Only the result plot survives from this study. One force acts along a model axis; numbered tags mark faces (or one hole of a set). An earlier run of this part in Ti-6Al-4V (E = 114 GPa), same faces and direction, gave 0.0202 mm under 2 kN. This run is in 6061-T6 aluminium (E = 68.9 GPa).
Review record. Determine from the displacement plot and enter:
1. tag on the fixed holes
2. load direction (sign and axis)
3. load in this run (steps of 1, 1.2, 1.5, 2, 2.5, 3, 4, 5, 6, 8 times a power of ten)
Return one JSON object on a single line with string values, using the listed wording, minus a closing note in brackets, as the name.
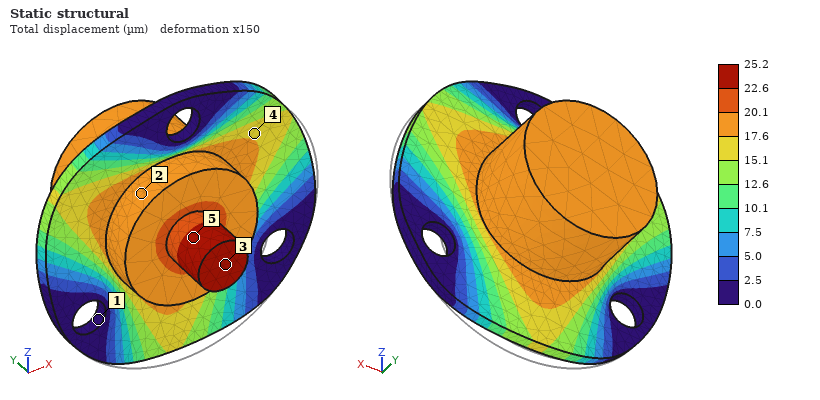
{"tag on the fixed holes": "1", "load direction": "+Y", "load in this run": "1.5 kN"}
